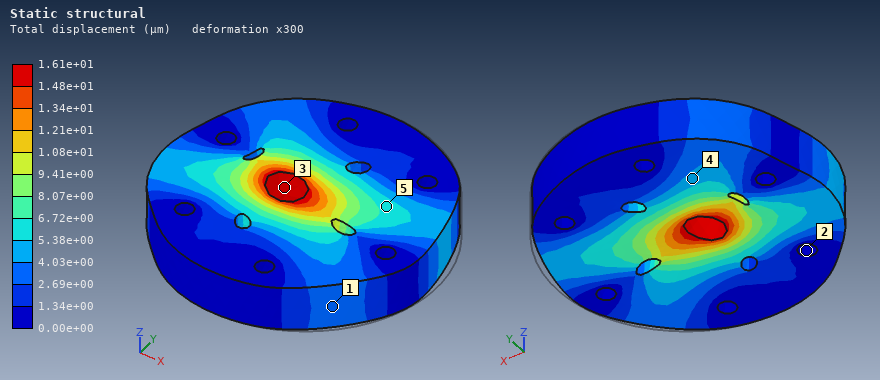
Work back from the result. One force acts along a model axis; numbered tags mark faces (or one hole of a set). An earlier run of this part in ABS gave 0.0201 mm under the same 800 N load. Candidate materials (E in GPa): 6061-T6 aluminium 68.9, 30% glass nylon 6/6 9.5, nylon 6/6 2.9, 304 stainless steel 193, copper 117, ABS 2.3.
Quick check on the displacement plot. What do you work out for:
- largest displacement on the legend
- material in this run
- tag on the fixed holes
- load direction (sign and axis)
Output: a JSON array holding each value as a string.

["1.61e+01 µm", "nylon 6/6", "2", "-X"]
